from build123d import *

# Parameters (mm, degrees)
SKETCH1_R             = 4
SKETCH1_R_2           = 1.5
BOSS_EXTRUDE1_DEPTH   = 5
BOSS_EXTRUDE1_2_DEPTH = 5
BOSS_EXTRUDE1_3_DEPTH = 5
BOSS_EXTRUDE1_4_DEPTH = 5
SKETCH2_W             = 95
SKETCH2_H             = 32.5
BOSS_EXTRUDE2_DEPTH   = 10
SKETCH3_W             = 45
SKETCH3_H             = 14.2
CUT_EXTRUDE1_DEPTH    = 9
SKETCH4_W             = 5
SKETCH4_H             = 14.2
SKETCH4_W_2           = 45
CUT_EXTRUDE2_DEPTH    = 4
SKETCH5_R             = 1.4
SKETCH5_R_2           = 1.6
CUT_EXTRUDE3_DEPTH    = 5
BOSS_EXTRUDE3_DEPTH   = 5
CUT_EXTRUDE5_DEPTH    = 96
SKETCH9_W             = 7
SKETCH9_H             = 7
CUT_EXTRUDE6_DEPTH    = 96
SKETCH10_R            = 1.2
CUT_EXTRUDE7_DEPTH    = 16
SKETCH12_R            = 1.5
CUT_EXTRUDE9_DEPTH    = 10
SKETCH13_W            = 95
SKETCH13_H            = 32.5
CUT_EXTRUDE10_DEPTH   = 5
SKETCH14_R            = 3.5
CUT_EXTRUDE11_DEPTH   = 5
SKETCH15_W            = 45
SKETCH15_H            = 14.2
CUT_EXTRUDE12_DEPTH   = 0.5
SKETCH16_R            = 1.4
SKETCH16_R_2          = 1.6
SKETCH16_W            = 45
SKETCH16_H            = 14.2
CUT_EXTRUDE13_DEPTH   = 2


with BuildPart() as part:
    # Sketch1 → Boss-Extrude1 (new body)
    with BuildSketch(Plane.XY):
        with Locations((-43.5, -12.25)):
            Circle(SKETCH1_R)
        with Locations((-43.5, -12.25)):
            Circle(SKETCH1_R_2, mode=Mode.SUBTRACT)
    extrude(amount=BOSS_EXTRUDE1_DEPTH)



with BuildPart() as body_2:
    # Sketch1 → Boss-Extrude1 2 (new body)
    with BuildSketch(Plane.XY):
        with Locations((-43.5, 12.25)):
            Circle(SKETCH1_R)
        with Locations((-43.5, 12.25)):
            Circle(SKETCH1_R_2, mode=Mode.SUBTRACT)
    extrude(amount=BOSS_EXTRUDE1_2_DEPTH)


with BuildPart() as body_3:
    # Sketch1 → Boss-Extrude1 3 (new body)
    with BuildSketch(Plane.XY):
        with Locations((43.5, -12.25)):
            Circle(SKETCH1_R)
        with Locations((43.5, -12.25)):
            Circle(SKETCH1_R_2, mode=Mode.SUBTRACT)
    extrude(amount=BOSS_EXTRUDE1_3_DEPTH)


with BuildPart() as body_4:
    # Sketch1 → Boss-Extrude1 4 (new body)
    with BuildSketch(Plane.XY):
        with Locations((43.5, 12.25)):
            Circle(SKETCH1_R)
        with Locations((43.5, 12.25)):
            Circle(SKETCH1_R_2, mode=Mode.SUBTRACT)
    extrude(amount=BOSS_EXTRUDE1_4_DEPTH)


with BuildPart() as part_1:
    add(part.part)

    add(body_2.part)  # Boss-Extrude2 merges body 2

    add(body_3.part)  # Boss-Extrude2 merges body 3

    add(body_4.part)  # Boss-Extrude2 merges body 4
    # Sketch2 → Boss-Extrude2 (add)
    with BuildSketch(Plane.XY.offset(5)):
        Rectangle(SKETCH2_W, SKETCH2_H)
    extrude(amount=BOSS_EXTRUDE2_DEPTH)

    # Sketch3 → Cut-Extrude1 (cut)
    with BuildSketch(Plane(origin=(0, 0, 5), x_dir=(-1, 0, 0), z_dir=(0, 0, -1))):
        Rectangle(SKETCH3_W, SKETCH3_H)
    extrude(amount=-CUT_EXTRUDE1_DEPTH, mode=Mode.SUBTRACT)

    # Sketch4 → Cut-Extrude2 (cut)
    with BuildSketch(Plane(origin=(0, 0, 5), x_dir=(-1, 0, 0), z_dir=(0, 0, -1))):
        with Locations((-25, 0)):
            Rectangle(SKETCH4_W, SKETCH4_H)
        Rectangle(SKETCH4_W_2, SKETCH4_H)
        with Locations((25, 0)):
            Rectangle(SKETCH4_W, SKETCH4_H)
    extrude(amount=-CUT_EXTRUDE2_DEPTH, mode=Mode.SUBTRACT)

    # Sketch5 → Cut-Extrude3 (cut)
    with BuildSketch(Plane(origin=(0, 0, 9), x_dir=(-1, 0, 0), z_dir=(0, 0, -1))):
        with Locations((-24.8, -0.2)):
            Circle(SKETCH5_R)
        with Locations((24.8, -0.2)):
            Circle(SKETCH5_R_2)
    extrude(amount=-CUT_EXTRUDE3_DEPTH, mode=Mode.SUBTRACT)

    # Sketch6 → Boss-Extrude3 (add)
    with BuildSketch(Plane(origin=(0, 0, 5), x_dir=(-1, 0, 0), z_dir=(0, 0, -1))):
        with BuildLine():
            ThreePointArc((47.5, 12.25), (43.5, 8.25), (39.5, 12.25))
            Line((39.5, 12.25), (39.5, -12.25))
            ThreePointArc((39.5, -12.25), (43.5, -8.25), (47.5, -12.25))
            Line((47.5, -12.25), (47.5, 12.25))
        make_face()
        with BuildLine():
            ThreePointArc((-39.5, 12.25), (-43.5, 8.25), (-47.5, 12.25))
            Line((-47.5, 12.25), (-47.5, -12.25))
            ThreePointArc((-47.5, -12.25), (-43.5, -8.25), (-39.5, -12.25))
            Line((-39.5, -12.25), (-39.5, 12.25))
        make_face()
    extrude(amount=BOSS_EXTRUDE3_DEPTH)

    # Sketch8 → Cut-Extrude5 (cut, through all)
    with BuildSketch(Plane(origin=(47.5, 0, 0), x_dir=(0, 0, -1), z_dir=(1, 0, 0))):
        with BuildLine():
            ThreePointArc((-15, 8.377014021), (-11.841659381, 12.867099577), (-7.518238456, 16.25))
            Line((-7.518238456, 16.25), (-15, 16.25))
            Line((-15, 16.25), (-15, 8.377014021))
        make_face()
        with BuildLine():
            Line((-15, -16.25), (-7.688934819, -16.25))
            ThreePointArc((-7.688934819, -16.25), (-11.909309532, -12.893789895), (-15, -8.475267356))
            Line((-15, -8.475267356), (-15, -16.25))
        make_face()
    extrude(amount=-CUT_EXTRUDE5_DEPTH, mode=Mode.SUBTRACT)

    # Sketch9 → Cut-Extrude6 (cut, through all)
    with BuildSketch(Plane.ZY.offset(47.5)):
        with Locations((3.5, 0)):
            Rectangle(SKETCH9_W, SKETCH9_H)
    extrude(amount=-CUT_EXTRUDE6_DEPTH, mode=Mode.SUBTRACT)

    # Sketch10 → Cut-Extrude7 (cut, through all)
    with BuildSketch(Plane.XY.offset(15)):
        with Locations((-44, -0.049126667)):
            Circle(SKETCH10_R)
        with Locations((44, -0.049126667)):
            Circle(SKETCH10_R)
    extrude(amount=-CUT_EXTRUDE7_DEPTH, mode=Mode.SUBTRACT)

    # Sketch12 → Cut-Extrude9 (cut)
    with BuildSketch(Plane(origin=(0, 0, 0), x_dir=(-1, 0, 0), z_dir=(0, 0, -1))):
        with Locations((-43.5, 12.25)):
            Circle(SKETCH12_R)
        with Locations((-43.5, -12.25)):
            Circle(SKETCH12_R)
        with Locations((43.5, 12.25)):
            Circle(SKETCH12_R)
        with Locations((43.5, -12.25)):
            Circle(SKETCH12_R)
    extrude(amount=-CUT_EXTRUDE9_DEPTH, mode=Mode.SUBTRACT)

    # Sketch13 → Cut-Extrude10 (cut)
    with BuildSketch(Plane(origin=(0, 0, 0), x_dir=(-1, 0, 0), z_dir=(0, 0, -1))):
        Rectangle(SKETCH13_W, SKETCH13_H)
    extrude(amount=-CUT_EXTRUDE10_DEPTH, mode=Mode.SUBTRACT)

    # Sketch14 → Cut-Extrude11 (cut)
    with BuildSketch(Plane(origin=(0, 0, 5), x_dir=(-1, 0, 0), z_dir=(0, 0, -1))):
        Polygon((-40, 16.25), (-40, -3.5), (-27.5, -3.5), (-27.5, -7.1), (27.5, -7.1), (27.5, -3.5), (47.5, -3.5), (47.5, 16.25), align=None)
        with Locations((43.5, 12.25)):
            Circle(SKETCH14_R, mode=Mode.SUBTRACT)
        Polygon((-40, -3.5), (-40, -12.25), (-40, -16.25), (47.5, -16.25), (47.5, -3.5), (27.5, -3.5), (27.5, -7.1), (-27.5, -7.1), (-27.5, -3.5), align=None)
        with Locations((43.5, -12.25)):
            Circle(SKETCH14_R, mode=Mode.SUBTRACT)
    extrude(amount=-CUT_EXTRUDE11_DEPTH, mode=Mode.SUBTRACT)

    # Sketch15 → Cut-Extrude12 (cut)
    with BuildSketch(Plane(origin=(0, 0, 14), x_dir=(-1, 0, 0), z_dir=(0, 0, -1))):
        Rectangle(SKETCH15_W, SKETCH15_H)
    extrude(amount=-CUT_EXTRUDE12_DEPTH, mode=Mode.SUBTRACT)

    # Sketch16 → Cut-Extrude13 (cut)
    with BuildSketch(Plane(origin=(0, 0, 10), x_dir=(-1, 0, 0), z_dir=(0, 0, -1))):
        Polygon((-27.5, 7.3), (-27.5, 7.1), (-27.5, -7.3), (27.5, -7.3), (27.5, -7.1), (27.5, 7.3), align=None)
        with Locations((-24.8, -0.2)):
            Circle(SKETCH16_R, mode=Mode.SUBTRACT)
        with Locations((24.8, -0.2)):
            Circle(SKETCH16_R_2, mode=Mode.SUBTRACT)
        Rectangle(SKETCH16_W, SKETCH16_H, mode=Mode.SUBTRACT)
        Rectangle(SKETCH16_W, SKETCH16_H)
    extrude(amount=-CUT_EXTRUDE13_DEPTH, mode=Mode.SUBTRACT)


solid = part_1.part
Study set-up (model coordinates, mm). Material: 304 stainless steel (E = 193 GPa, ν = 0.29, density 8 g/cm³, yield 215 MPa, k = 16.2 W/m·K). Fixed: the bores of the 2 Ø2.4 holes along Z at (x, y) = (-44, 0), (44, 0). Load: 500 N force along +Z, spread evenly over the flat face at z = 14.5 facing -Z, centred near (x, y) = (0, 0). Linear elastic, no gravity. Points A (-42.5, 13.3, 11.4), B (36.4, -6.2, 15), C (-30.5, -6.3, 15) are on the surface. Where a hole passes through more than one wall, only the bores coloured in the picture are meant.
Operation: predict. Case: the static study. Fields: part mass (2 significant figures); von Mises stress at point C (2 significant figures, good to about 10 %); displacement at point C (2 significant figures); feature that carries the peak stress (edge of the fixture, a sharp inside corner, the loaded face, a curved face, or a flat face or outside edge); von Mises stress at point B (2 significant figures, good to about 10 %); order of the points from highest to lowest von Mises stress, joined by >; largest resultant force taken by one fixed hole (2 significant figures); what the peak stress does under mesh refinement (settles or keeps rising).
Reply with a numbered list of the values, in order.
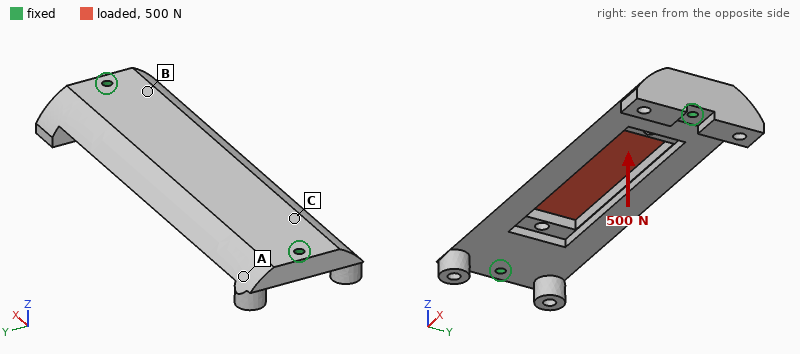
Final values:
1. 75 g
2. 21 MPa
3. 14 µm
4. edge of the fixture
5. 41 MPa
6. B > C > A
7. 260 N
8. keeps rising
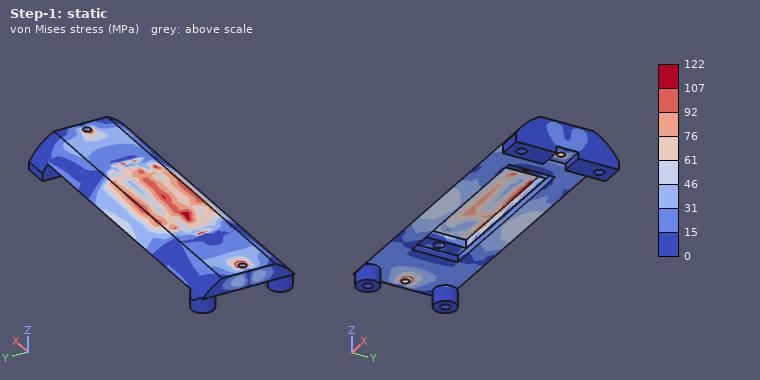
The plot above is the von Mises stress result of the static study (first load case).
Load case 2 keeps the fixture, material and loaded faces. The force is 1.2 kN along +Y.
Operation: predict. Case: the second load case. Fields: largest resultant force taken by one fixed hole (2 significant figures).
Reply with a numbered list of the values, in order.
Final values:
1. 620 N
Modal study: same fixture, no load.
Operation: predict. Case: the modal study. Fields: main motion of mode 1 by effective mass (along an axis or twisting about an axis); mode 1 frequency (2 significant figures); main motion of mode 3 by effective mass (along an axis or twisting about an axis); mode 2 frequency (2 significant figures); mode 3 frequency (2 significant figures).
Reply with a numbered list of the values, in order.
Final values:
1. along Z
2. 3600 Hz
3. along Y
4. 4600 Hz
5. 8000 Hz
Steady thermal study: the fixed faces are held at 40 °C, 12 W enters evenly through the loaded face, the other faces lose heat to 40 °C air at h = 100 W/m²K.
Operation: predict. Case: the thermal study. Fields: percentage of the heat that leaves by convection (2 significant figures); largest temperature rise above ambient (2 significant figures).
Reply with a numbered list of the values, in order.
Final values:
1. 88 %
2. 74 K
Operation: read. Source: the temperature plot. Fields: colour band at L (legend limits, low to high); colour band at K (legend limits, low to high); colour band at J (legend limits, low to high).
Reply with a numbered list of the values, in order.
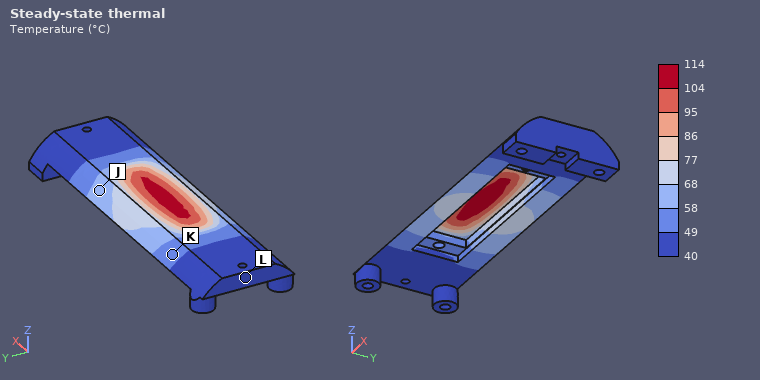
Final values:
1. 40 to 49 °C
2. 49 to 58 °C
3. 58 to 68 °C
